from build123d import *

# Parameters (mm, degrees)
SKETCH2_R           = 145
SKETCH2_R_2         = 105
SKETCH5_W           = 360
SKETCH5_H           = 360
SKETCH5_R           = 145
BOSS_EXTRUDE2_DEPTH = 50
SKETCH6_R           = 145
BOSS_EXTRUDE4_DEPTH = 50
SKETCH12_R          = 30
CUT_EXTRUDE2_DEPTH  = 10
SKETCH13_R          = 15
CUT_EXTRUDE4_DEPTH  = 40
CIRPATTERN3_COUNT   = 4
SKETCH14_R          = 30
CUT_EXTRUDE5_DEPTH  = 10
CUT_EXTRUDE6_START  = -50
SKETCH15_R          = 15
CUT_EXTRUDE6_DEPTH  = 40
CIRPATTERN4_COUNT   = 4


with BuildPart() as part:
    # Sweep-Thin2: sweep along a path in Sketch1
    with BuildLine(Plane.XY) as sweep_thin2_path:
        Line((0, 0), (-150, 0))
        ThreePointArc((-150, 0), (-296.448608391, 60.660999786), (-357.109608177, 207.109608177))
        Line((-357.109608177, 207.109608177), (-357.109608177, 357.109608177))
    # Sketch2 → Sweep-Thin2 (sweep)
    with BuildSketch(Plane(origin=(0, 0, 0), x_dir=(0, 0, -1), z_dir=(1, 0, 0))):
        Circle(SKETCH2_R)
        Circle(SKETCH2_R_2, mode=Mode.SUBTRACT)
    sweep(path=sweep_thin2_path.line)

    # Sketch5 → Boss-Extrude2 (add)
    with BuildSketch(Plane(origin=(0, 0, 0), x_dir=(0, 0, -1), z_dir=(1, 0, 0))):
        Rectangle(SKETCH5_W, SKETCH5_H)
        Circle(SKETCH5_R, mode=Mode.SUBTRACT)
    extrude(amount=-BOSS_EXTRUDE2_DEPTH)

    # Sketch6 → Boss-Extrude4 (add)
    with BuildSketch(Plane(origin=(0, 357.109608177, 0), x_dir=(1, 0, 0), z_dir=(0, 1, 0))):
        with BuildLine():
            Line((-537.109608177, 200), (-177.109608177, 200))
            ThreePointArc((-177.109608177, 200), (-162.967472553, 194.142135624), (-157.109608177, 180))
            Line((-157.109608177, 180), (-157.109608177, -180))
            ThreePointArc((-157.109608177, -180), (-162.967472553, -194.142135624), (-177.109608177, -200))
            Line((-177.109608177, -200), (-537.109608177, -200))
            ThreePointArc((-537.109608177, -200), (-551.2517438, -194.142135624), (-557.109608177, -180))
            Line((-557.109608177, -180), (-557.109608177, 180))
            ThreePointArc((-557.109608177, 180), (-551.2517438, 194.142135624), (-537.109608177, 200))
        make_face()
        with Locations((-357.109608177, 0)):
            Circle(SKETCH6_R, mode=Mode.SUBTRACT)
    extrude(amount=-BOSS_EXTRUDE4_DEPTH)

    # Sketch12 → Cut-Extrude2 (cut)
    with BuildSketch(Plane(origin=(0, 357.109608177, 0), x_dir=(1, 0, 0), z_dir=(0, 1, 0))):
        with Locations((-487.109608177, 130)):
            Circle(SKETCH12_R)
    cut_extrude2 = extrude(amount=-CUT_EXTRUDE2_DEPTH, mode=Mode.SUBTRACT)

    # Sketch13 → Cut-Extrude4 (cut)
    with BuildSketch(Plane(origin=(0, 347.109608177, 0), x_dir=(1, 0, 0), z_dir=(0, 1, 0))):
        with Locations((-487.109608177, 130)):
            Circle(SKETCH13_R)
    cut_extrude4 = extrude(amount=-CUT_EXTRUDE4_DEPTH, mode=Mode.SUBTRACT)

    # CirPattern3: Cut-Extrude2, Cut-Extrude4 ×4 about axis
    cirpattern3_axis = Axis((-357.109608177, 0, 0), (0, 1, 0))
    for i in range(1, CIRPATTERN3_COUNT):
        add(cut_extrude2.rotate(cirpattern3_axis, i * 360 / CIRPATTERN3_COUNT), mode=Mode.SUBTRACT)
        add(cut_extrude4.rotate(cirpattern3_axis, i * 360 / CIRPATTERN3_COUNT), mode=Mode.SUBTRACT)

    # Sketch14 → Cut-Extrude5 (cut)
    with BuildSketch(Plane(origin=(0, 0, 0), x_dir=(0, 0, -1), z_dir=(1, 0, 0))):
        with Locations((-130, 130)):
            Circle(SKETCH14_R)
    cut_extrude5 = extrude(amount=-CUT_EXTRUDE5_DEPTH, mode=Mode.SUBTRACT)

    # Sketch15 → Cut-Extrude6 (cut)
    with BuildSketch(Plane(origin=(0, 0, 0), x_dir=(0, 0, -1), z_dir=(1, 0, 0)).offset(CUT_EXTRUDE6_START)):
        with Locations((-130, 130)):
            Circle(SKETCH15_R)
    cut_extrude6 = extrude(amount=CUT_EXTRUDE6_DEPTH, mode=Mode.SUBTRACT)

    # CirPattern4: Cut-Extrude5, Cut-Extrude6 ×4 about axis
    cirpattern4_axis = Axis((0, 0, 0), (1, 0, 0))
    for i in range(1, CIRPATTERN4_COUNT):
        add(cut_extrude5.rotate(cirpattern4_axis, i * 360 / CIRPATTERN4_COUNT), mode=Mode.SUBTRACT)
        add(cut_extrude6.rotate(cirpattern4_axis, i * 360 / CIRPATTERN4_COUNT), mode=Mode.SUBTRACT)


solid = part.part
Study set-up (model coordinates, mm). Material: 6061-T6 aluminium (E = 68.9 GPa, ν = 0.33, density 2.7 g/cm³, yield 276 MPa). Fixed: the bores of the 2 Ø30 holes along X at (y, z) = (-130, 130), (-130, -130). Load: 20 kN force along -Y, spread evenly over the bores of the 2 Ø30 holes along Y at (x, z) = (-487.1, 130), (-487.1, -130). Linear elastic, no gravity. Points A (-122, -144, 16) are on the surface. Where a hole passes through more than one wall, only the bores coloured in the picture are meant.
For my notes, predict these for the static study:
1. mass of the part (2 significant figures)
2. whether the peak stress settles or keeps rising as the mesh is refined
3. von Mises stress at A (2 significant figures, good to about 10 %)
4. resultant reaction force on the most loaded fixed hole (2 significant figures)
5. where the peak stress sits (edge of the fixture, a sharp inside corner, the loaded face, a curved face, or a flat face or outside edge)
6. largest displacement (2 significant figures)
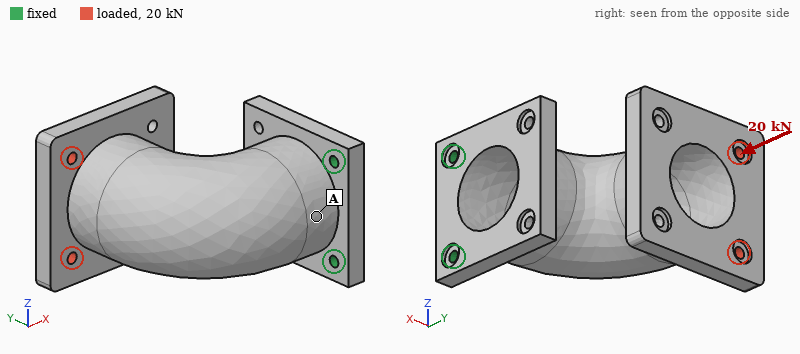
73 kg
keeps rising
12 MPa
10 kN
edge of the fixture
2.6 mm
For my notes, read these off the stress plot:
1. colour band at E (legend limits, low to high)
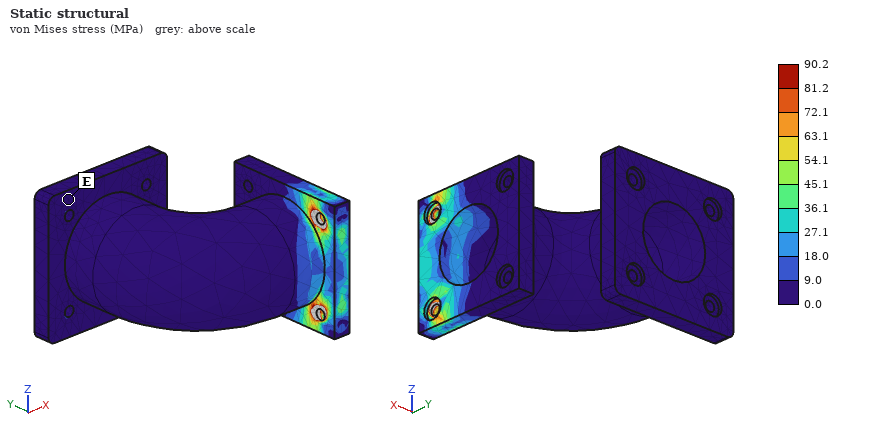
0.0 to 9.0 MPa
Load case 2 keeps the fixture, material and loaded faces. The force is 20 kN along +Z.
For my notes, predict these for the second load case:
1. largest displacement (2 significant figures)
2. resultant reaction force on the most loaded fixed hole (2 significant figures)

0.40 mm
51 kN
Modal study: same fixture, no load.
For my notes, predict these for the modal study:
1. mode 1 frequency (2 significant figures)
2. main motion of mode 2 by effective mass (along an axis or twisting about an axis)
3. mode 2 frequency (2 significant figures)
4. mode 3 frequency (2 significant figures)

75 Hz
along Z
240 Hz
530 Hz
